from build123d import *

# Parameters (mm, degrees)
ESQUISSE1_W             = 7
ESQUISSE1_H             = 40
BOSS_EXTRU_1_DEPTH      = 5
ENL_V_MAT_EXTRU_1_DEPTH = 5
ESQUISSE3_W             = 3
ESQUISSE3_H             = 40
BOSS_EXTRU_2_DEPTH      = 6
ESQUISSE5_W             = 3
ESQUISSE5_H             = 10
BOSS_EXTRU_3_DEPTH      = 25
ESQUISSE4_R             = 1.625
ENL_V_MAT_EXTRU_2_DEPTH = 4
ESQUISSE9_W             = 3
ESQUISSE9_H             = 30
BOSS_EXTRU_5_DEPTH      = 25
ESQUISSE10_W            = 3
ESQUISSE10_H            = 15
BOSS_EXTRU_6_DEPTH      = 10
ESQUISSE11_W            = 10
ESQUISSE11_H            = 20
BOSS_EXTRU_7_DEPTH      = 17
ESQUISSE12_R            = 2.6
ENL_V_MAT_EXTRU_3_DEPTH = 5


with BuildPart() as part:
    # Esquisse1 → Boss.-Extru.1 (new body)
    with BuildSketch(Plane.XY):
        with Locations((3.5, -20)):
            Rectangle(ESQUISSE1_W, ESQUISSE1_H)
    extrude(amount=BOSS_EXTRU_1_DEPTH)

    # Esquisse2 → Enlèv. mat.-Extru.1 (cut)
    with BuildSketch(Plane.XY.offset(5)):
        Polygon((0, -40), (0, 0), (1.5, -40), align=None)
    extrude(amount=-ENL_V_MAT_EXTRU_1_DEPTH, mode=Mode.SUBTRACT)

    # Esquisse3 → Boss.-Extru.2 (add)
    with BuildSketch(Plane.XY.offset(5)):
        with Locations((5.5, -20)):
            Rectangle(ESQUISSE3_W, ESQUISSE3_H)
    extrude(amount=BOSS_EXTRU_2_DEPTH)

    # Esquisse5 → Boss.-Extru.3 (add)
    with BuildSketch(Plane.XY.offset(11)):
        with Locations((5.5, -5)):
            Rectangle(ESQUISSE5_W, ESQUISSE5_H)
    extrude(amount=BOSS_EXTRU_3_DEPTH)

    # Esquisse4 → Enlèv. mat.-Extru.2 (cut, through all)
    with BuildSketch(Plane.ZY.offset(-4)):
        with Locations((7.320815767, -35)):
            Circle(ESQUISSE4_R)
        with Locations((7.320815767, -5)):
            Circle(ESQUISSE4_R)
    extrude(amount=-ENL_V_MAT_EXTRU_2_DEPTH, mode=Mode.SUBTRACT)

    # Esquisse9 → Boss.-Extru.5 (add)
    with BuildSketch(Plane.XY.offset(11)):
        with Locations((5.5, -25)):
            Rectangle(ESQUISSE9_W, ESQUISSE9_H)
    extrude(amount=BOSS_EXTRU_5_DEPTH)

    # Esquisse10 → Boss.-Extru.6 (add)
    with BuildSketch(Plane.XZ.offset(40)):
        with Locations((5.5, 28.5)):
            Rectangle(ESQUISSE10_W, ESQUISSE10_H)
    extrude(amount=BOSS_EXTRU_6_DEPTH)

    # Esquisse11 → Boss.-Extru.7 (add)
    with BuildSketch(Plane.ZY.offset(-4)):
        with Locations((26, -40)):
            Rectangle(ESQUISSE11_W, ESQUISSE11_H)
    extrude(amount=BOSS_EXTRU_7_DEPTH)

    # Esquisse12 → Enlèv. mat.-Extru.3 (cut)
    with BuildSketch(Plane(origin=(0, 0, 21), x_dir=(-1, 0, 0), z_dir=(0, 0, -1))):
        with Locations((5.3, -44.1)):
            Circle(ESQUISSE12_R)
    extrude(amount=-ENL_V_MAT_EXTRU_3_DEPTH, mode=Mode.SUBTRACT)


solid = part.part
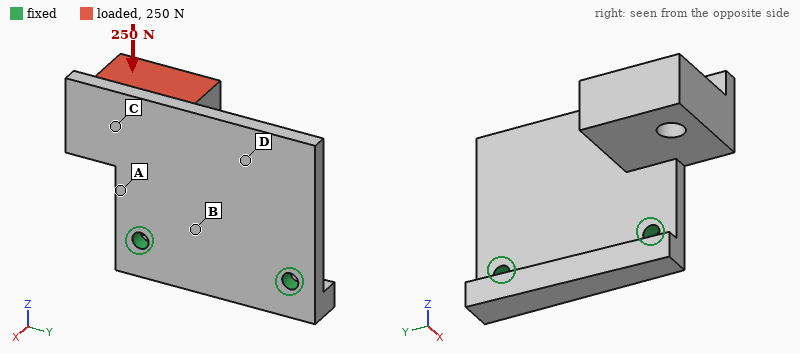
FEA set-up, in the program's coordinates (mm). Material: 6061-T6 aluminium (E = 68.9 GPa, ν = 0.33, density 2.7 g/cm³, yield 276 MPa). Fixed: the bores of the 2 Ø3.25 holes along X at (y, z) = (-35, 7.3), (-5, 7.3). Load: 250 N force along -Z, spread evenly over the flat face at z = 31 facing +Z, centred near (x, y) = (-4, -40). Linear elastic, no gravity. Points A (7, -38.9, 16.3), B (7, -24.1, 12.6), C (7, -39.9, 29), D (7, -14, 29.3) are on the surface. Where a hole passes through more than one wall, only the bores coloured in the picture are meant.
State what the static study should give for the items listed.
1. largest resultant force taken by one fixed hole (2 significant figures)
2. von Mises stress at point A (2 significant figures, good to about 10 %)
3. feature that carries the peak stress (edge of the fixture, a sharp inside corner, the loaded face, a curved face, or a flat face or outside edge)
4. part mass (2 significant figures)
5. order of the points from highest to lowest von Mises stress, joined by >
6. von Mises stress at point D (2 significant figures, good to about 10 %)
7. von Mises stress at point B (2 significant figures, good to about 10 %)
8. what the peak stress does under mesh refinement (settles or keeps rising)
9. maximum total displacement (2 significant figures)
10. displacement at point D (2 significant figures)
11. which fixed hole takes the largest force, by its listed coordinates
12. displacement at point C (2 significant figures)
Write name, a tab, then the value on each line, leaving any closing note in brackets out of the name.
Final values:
largest resultant force taken by one fixed hole	290 N
von Mises stress at point A	60 MPa
feature that carries the peak stress	edge of the fixture
part mass	23 g
order of the points from highest to lowest von Mises stress, joined by >	A > B > D > C
von Mises stress at point D	21 MPa
von Mises stress at point B	34 MPa
what the peak stress does under mesh refinement	keeps rising
maximum total displacement	0.23 mm
displacement at point D	0.087 mm
which fixed hole takes the largest force, by its listed coordinates	(-35, 7.3)
displacement at point C	0.13 mm
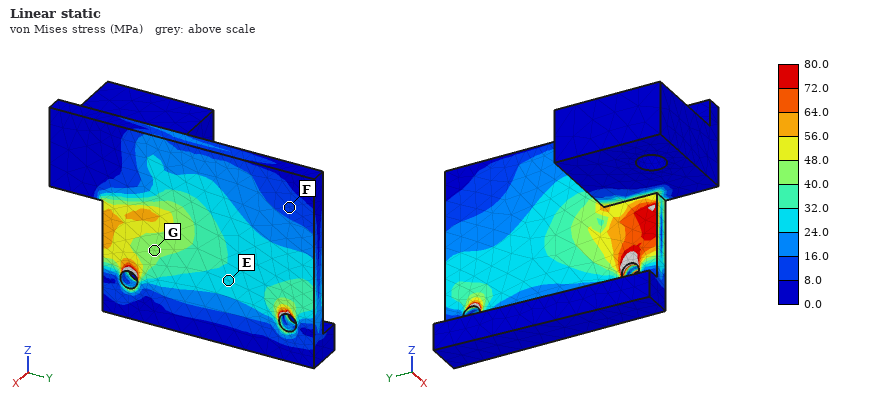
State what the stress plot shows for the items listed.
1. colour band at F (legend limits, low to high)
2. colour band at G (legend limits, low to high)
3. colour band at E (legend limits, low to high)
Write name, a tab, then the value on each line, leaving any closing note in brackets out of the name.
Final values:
colour band at F	8.0 to 16.0 MPa
colour band at G	40.0 to 48.0 MPa
colour band at E	24.0 to 32.0 MPa
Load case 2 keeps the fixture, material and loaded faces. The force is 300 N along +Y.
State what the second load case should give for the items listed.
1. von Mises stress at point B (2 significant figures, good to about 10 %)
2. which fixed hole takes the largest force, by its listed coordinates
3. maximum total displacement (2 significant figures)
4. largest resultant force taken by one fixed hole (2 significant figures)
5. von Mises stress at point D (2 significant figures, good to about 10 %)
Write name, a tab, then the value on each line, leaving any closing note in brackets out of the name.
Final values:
von Mises stress at point B	16 MPa
which fixed hole takes the largest force, by its listed coordinates	(-5, 7.3)
maximum total displacement	0.16 mm
largest resultant force taken by one fixed hole	300 N
von Mises stress at point D	13 MPa
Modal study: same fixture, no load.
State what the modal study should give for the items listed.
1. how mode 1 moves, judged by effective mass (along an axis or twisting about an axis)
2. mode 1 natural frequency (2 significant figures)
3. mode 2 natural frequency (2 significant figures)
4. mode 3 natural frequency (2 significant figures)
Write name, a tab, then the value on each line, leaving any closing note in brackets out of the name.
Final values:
how mode 1 moves, judged by effective mass	along X
mode 1 natural frequency	1400 Hz
mode 2 natural frequency	2500 Hz
mode 3 natural frequency	5400 Hz
